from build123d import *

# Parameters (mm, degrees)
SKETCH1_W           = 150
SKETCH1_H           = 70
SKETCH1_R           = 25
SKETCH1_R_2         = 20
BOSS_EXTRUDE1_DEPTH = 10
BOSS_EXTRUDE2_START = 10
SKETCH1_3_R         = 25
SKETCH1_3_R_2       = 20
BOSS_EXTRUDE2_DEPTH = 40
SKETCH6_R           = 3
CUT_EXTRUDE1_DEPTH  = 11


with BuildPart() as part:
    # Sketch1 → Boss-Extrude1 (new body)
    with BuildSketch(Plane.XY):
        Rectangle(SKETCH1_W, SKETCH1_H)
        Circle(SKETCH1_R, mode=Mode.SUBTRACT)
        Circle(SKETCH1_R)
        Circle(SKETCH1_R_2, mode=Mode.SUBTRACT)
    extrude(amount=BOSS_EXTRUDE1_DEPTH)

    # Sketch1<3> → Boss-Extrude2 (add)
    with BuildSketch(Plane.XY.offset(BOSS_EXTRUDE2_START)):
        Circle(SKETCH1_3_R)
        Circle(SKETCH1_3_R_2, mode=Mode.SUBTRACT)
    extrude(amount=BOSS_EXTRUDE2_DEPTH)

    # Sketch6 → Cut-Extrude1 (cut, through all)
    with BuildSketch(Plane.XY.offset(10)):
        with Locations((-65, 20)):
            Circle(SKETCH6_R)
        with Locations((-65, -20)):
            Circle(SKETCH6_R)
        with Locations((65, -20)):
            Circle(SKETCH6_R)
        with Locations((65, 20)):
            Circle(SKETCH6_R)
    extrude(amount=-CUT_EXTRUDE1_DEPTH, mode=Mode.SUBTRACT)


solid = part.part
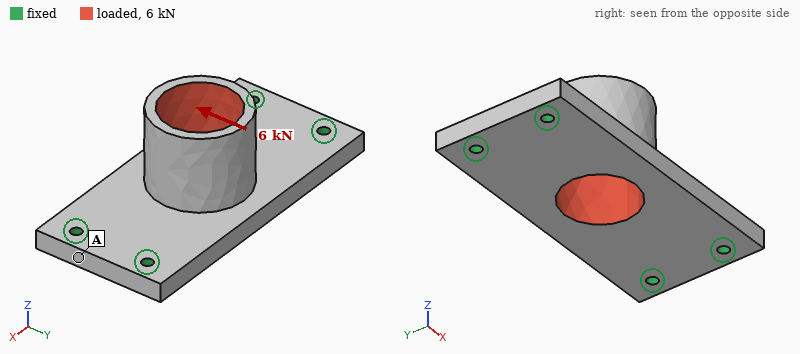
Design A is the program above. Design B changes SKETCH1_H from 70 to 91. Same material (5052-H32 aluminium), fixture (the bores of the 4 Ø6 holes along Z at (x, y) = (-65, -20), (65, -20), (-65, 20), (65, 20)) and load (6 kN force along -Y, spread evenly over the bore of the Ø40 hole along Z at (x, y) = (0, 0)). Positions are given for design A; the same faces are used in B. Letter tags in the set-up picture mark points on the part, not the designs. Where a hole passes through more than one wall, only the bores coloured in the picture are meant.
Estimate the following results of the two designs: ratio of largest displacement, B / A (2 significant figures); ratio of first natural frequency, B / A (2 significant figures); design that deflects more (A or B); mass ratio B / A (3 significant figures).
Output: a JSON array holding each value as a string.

["0.80", "0.96", "A", "1.26"]
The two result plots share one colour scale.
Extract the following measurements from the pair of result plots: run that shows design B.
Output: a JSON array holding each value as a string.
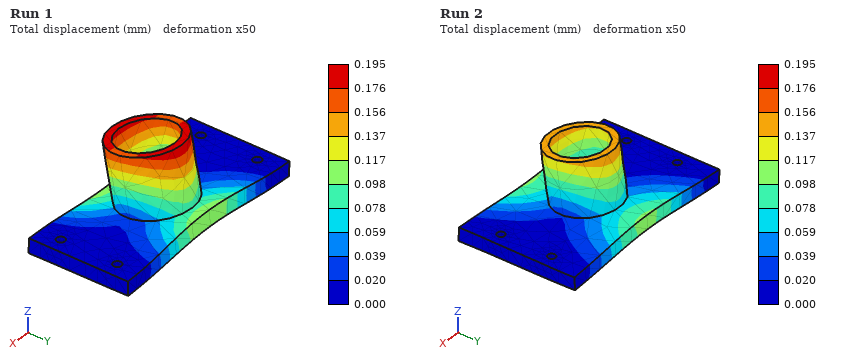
["Run 2"]
